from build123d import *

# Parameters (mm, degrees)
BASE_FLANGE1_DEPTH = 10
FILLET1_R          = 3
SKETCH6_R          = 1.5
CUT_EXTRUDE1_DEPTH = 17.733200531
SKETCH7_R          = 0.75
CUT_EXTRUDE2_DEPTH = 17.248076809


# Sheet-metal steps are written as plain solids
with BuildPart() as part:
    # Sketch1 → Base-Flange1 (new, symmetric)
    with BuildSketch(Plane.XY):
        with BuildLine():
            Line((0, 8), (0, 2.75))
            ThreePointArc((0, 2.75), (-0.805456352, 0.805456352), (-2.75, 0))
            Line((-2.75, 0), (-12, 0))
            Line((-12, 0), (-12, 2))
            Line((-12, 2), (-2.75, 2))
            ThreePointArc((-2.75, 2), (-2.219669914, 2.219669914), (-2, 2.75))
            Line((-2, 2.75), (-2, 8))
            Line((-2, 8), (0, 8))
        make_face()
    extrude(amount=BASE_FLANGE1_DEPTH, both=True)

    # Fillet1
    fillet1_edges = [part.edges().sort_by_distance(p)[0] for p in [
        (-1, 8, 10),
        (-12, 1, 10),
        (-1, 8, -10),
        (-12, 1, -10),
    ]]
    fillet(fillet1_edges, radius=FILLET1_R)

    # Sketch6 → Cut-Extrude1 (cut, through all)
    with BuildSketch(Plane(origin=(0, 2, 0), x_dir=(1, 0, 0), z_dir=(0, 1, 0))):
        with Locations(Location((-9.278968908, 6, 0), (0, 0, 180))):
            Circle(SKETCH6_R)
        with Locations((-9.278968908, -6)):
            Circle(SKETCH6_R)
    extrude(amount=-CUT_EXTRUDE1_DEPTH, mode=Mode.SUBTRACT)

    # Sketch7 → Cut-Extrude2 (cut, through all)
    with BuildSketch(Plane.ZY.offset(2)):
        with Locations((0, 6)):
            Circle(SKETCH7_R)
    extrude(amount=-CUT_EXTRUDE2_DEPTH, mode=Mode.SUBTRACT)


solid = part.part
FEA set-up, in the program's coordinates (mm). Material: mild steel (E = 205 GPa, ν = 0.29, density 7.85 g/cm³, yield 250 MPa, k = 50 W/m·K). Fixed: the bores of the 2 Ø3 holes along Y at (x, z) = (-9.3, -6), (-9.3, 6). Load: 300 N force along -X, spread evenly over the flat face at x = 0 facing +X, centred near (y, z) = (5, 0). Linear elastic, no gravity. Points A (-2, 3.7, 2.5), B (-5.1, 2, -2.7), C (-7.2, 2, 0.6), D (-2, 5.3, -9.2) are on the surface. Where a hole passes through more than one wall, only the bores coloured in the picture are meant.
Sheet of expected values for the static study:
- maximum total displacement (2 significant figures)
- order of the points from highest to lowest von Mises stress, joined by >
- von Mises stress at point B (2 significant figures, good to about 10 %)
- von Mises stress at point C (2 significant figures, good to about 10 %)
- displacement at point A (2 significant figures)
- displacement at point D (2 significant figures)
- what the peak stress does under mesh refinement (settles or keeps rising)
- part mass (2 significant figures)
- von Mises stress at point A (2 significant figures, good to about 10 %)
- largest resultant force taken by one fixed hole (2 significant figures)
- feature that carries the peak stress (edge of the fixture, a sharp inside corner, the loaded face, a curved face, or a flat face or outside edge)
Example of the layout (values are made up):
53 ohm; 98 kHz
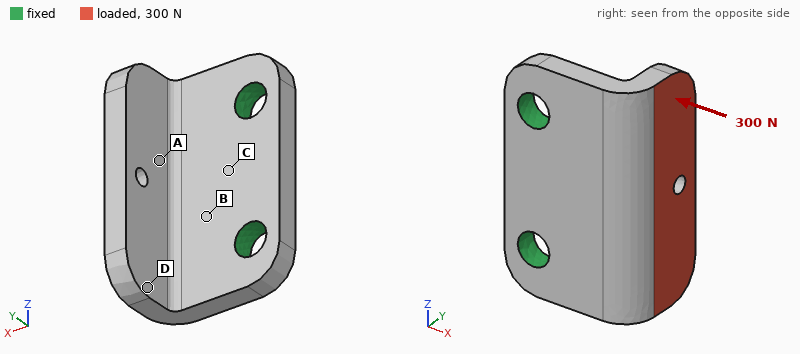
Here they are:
33 µm; B > C > A > D; 89 MPa; 63 MPa; 14 µm; 19 µm; keeps rising; 5.0 g; 36 MPa; 150 N; edge of the fixture
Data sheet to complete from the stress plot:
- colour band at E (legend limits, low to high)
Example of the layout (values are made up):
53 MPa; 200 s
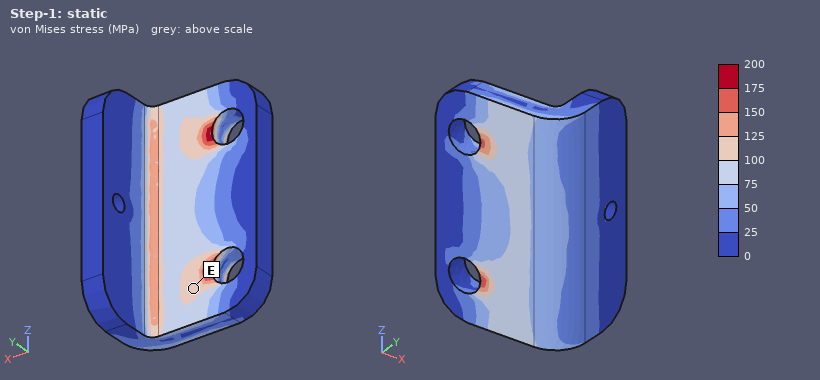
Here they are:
100 to 125 MPa
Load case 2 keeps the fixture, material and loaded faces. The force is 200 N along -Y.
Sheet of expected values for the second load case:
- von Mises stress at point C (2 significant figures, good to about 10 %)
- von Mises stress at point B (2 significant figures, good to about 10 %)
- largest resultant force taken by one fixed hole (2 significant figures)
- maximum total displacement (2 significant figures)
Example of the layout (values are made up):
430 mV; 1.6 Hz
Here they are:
59 MPa; 64 MPa; 100 N; 26 µm
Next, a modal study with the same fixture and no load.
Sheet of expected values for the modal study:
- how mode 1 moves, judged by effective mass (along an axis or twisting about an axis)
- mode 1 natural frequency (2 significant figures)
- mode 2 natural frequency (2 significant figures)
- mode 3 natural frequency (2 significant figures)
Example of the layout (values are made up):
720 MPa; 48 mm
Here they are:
along Y; 11 kHz; 17 kHz; 31 kHz
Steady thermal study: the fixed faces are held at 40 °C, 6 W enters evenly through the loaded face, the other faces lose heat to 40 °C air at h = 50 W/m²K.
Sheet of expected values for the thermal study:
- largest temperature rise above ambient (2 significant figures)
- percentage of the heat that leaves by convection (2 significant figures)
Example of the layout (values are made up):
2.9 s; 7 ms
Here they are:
34 K; 8.6 %
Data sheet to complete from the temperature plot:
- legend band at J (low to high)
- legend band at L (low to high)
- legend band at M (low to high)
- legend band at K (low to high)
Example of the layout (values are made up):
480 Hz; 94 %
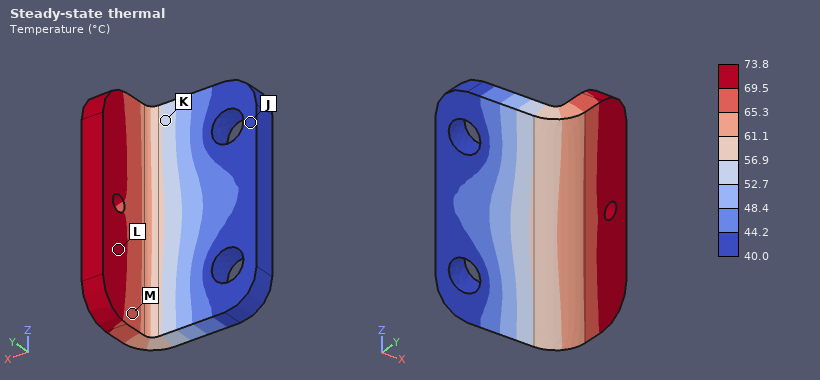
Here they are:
40.0 to 44.2 °C; 69.5 to 73.8 °C; 65.3 to 69.5 °C; 52.7 to 56.9 °C
